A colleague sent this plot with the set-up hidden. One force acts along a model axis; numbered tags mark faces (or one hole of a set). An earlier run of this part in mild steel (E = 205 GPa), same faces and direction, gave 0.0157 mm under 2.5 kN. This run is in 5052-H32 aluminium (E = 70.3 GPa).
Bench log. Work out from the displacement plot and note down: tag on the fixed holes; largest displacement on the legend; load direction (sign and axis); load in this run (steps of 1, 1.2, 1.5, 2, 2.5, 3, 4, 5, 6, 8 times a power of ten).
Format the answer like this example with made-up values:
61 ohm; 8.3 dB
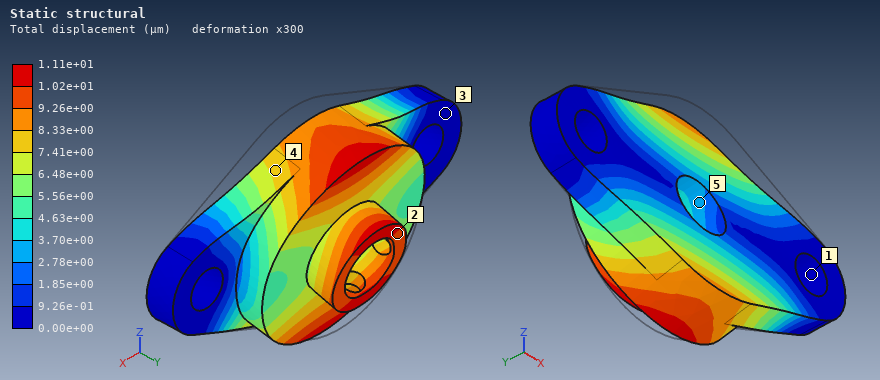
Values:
1; 1.11e+01 µm; -Z; 600 N
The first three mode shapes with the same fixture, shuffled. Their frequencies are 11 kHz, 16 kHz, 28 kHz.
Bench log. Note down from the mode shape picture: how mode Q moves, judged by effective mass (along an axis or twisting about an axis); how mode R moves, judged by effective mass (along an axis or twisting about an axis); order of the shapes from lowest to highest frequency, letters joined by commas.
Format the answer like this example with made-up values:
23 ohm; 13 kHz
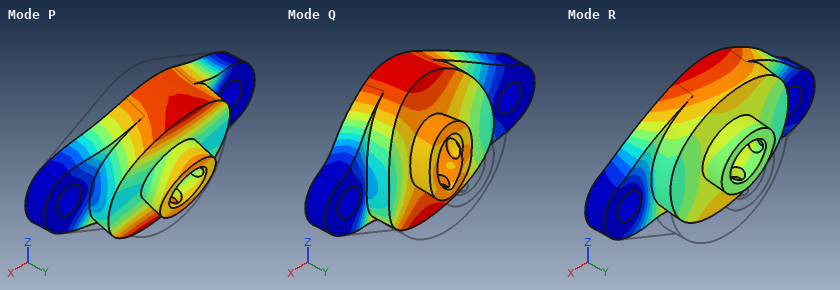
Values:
along Y; along Z; P, Q, R
